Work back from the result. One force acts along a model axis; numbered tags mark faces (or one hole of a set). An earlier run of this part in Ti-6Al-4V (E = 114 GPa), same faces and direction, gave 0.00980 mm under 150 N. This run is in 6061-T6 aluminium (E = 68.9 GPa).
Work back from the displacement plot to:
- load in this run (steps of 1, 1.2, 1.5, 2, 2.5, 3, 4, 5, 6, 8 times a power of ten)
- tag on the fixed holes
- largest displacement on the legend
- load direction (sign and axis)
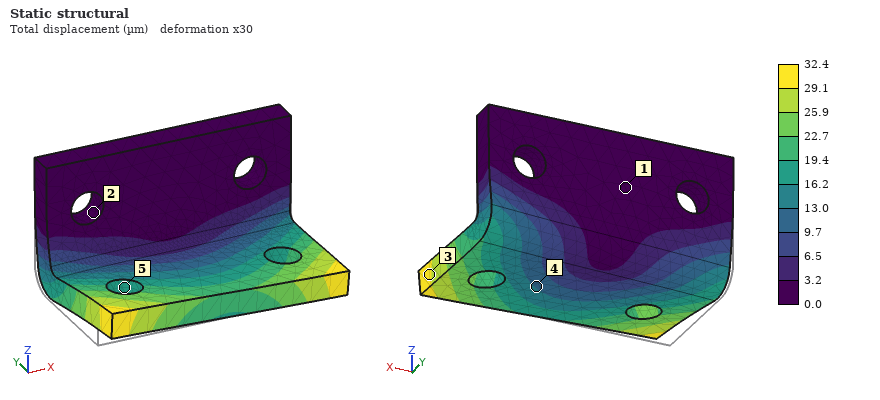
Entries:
300 N
2
32.4 µm
+X
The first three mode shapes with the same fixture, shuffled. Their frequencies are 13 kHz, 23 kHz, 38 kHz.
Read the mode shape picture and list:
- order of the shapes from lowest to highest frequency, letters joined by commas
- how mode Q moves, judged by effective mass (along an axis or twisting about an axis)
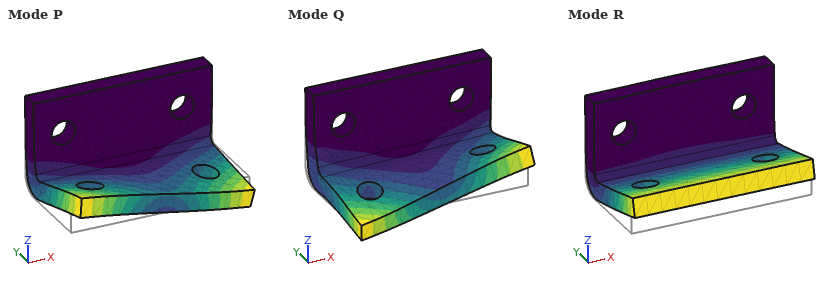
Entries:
R, P, Q
along X
